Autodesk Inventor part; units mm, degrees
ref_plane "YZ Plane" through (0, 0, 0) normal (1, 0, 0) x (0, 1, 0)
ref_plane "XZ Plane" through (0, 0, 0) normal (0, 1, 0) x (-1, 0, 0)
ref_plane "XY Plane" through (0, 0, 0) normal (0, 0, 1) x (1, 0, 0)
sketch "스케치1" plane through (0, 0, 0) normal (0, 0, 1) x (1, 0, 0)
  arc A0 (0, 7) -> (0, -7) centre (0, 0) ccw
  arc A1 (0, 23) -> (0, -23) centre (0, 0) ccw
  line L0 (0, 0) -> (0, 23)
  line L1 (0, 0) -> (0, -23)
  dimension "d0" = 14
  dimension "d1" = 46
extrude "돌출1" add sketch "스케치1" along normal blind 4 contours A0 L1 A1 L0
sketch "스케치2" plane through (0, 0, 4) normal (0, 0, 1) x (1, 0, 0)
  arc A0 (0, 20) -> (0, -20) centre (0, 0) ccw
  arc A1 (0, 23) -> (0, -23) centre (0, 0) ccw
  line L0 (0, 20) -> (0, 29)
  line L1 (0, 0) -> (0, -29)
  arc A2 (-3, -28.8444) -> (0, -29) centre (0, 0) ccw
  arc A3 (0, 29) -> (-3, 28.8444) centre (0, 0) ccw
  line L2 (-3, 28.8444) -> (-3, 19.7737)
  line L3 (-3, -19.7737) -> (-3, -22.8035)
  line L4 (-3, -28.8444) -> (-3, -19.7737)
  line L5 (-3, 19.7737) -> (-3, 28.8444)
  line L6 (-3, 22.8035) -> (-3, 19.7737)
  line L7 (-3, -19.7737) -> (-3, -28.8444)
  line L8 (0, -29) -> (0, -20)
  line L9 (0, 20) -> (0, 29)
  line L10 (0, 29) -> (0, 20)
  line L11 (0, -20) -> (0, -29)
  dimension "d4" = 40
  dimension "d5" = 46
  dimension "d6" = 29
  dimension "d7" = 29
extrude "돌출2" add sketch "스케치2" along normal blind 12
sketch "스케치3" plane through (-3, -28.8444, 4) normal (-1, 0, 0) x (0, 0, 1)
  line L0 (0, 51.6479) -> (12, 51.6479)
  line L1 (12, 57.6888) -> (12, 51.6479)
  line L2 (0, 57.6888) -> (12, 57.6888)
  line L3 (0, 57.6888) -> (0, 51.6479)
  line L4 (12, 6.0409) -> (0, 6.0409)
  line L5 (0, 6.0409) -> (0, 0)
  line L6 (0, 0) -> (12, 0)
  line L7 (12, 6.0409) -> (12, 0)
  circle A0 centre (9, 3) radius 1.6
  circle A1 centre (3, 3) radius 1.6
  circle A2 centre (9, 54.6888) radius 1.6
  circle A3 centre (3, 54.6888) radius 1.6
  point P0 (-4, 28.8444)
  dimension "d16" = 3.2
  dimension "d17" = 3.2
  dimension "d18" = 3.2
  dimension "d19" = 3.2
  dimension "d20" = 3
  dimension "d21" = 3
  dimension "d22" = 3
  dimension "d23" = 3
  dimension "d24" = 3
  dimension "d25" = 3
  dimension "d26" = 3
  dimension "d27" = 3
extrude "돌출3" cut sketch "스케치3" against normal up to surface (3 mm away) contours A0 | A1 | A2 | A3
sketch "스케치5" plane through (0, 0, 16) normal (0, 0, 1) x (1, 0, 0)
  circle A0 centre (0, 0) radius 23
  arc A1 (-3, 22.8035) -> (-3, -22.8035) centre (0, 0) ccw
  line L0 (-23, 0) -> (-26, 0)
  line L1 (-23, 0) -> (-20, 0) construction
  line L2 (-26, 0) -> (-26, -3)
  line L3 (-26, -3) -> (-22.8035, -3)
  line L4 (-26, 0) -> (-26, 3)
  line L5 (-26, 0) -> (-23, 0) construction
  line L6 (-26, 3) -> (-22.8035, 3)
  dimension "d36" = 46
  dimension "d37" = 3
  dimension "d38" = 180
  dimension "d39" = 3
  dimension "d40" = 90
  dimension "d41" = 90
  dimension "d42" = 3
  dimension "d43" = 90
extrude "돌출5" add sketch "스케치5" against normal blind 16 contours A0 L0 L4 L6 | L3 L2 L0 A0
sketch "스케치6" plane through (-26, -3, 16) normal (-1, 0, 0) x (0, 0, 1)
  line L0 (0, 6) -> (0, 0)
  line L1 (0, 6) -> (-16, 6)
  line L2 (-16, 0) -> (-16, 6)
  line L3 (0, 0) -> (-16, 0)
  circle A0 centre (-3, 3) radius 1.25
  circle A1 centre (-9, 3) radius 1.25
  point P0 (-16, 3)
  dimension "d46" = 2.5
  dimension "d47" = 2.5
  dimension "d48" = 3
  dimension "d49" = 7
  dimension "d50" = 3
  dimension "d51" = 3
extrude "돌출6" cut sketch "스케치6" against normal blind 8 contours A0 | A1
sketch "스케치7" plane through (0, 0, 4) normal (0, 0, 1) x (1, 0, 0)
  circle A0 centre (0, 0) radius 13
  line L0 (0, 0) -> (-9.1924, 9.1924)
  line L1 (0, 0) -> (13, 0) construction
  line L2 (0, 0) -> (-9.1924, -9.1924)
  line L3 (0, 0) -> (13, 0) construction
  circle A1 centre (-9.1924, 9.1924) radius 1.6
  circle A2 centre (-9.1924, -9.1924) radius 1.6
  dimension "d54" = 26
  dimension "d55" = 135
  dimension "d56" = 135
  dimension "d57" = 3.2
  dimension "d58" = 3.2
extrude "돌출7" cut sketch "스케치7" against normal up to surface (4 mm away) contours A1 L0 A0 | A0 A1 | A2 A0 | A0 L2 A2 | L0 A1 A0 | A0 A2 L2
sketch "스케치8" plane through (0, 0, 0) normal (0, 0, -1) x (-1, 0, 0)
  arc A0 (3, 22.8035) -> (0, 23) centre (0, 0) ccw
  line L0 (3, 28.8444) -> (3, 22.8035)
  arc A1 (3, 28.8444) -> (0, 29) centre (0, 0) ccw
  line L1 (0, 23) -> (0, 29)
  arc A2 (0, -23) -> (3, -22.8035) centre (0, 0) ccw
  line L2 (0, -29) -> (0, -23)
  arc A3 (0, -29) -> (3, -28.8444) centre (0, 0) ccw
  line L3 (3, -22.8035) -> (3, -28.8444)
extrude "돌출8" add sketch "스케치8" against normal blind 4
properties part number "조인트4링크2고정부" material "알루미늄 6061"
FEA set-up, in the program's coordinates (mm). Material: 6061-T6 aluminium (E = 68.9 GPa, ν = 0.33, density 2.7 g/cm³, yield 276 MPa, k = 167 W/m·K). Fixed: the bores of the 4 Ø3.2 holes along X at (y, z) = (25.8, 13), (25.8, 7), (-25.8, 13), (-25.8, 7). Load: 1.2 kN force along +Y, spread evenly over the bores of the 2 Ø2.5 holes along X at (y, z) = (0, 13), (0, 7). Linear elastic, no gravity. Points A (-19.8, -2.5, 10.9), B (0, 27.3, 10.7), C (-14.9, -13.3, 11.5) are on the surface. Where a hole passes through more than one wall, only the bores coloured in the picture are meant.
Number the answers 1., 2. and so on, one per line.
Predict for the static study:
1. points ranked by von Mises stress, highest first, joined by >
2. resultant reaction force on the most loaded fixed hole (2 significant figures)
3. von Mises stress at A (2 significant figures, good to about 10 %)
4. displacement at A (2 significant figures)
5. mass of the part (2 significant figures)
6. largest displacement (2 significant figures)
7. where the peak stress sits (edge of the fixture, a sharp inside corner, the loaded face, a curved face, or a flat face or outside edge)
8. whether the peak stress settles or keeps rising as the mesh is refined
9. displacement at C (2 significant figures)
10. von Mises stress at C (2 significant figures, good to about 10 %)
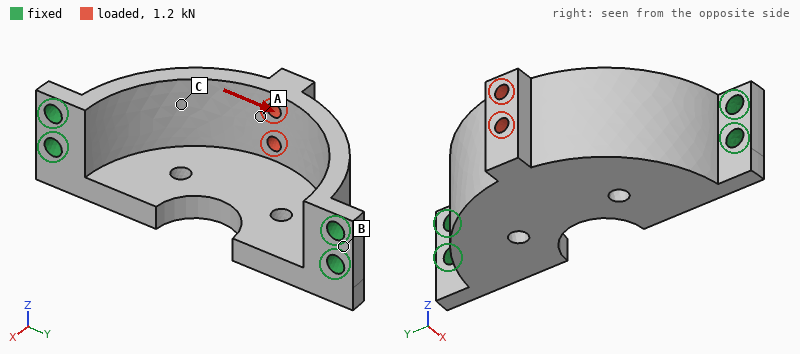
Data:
1. C > A > B
2. 800 N
3. 25 MPa
4. 29 µm
5. 16 g
6. 46 µm
7. edge of the fixture
8. keeps rising
9. 31 µm
10. 42 MPa
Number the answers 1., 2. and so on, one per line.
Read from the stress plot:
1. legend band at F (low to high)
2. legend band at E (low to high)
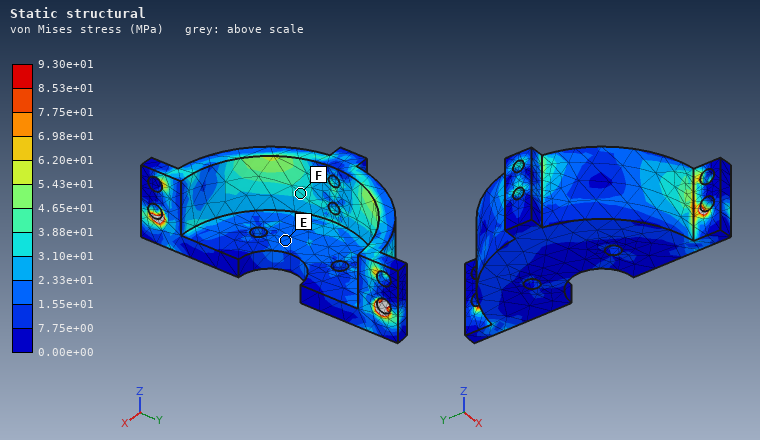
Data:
1. 3.10e+01 to 3.88e+01 MPa
2. 1.55e+01 to 2.33e+01 MPa
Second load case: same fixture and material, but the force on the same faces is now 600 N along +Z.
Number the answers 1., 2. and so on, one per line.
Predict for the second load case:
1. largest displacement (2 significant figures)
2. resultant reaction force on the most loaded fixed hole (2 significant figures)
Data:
1. 0.10 mm
2. 850 N
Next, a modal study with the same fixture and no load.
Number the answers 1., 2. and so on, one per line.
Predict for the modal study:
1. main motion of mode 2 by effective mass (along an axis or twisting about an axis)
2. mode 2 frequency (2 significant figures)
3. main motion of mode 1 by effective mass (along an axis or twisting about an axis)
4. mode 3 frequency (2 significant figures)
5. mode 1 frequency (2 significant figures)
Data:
1. along Y
2. 11 kHz
3. along Z
4. 15 kHz
5. 5700 Hz
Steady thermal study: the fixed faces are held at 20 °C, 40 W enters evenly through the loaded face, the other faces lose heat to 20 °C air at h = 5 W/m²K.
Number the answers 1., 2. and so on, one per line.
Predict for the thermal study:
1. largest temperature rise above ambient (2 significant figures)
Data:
1. 70 K
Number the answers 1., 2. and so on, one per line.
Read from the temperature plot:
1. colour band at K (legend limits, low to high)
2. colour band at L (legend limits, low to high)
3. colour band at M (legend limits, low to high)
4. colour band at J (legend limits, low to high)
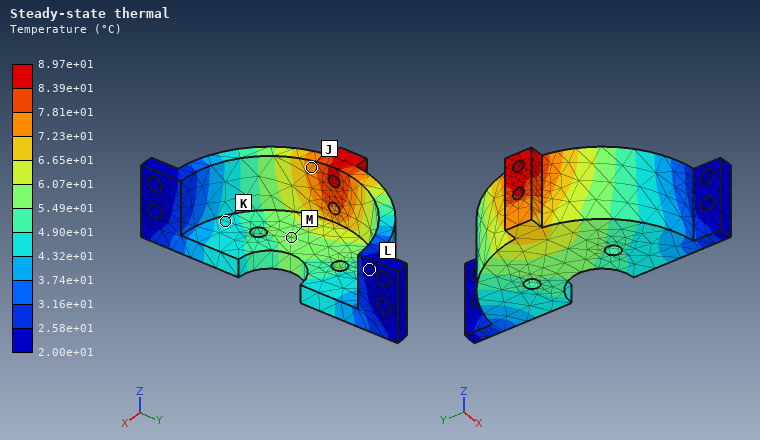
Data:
1. 4.32e+01 to 4.90e+01 °C
2. 2.00e+01 to 2.58e+01 °C
3. 5.49e+01 to 6.07e+01 °C
4. 7.23e+01 to 7.81e+01 °C
